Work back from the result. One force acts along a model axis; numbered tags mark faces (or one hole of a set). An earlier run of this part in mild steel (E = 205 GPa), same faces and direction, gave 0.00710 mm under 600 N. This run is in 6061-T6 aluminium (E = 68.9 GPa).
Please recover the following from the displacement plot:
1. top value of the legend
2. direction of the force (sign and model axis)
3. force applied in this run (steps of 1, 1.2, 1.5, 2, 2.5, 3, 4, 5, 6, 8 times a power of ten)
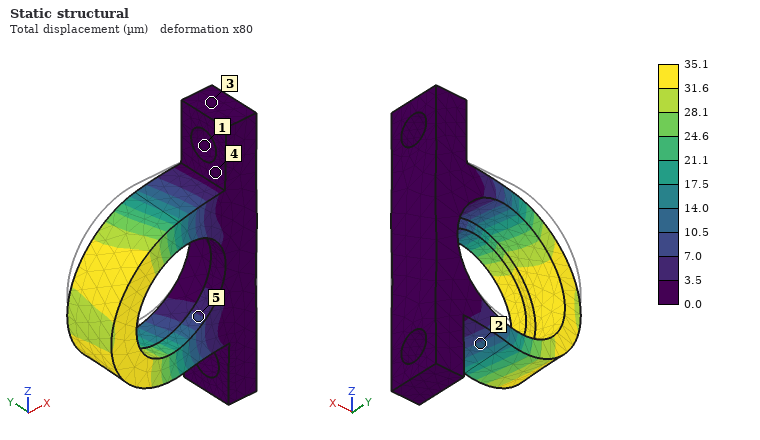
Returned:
35.1 µm
-Z
1 kN
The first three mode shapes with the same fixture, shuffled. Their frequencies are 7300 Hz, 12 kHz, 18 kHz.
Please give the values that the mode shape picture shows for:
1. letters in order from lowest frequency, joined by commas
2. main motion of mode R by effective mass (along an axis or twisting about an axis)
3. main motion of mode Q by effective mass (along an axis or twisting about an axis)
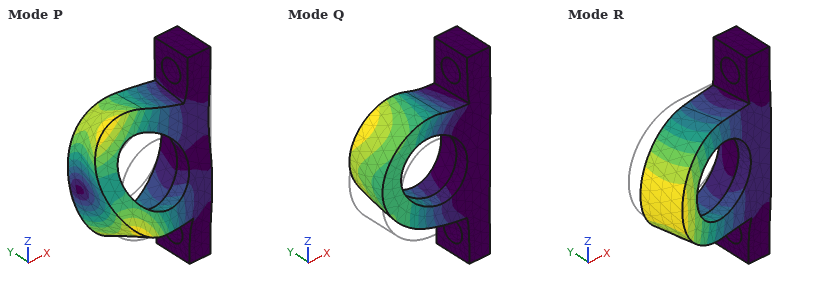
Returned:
R, Q, P
along Y
along Z
